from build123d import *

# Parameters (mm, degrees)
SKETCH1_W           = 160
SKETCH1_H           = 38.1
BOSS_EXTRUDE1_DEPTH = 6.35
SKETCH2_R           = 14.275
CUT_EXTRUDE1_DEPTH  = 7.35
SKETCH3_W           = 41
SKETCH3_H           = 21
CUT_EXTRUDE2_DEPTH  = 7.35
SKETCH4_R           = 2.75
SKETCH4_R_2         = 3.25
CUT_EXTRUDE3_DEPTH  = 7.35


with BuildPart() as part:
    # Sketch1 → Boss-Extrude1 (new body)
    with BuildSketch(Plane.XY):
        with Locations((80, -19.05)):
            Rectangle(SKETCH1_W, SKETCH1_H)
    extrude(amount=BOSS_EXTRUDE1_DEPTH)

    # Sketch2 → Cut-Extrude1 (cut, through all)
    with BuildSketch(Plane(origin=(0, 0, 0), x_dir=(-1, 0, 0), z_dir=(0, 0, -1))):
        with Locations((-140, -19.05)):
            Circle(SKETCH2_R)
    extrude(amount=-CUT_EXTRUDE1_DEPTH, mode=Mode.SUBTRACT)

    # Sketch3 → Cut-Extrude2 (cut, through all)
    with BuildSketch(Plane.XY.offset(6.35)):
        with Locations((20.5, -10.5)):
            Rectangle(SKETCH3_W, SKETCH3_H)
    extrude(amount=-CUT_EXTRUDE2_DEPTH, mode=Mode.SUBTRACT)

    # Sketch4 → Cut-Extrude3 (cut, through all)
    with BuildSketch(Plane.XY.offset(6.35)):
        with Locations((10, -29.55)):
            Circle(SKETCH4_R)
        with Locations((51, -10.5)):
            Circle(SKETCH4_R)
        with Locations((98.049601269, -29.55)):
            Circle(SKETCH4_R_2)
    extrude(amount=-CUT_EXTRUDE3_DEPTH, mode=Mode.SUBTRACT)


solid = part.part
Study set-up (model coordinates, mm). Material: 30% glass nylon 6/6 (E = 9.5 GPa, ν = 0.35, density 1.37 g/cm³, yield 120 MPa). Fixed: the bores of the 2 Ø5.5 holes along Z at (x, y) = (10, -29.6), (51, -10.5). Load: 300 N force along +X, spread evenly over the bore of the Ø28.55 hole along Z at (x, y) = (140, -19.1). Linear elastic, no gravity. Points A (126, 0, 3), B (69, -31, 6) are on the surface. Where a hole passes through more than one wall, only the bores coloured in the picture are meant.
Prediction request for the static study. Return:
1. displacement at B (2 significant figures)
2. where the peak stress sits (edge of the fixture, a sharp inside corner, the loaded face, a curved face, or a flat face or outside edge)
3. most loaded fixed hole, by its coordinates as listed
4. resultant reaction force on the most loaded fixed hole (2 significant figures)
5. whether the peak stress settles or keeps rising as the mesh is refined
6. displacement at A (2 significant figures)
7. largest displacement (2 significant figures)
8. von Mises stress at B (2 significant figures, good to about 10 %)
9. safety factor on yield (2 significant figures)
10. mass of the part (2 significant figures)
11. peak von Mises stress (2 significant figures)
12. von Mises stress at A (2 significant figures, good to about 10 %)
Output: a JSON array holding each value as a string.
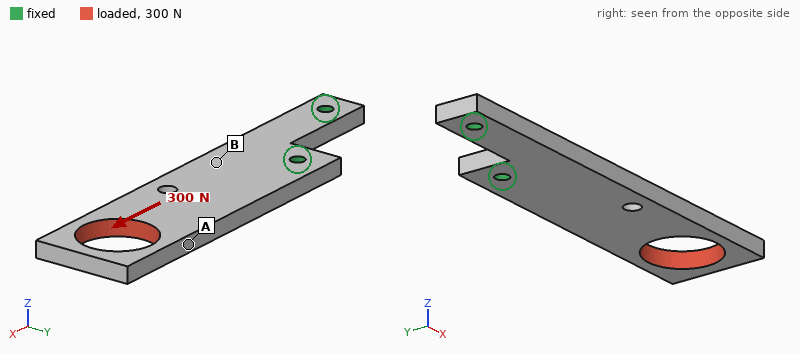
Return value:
["7.7 µm", "the loaded face", "(51, -10.5)", "200 N", "settles", "16 µm", "42 µm", "1.2 MPa", "17", "39 g", "7.1 MPa", "4.0 MPa"]
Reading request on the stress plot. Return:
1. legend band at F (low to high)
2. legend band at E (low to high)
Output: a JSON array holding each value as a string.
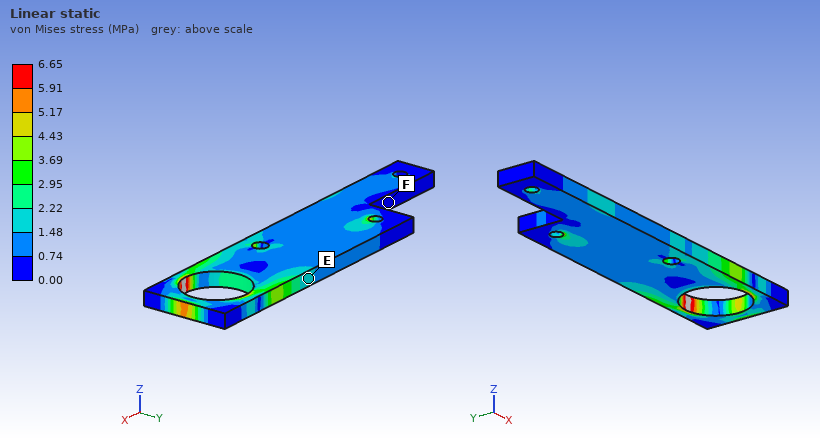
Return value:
["0.00 to 0.74 MPa", "1.48 to 2.22 MPa"]
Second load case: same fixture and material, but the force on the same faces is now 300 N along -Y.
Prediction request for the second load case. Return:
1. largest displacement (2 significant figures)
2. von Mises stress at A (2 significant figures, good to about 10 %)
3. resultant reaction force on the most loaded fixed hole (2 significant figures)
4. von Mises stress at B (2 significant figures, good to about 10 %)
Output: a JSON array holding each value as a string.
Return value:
["0.74 mm", "12 MPa", "990 N", "8.8 MPa"]
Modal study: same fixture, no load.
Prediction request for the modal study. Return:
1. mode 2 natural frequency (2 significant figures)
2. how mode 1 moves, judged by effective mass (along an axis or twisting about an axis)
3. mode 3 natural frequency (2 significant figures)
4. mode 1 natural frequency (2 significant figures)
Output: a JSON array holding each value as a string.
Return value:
["1100 Hz", "along Z", "1100 Hz", "270 Hz"]
